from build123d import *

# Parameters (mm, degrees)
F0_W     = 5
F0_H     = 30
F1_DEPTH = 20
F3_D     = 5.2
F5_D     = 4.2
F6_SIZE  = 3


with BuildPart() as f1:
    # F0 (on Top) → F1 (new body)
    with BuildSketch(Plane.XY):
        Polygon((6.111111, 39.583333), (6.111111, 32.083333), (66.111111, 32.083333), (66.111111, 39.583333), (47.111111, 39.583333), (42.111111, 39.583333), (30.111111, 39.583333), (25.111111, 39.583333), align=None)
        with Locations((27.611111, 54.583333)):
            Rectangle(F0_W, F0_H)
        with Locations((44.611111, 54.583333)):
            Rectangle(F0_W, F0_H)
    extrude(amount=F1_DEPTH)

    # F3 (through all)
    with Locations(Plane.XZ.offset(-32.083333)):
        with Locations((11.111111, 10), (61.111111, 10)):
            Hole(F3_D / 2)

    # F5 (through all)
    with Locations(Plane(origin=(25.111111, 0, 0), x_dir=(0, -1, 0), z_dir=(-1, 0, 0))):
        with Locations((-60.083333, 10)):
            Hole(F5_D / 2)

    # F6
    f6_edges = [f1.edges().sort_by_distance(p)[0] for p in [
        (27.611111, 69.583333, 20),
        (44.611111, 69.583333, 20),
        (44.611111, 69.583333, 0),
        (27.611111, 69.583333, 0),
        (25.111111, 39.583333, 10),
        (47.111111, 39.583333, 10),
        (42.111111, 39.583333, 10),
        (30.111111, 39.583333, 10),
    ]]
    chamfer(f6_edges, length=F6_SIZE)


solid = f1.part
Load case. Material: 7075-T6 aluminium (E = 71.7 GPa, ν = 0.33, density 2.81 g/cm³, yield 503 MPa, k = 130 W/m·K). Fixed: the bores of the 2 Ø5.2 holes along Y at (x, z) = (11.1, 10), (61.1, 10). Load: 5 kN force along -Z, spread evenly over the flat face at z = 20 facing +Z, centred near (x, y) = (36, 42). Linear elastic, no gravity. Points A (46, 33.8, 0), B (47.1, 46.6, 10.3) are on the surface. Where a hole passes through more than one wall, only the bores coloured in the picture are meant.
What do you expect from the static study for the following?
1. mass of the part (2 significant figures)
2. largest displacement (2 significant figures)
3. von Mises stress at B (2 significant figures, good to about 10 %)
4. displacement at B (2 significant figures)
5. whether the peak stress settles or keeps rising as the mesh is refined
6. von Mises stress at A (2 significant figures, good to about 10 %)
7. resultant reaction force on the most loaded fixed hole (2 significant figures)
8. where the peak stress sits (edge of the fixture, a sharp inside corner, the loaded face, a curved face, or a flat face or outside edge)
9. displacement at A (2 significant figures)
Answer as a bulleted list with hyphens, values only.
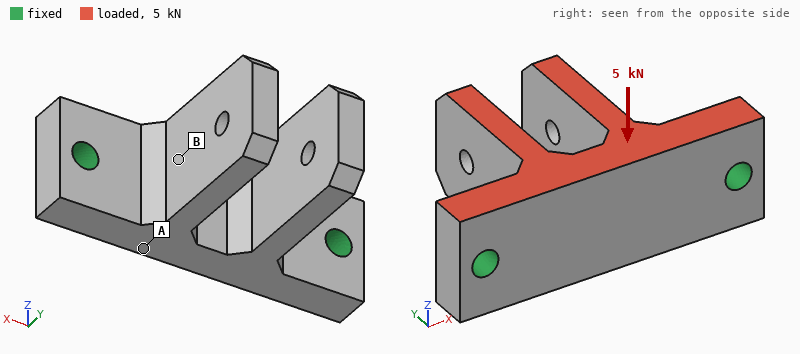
- 42 g
- 0.15 mm
- 22 MPa
- 0.055 mm
- keeps rising
- 47 MPa
- 2.5 kN
- edge of the fixture
- 0.033 mm
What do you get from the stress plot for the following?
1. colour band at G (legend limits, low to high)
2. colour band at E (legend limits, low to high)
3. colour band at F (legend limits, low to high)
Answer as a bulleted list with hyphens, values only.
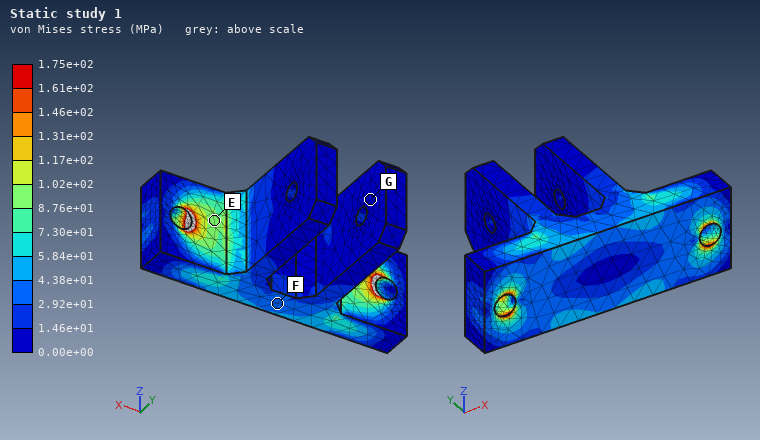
- 0.00e+00 to 1.46e+01 MPa
- 8.76e+01 to 1.02e+02 MPa
- 2.92e+01 to 4.38e+01 MPa
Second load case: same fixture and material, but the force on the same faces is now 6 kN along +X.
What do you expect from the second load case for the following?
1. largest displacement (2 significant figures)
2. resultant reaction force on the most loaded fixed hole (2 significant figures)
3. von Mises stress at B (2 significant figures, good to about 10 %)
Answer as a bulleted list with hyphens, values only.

- 0.23 mm
- 3.3 kN
- 110 MPa
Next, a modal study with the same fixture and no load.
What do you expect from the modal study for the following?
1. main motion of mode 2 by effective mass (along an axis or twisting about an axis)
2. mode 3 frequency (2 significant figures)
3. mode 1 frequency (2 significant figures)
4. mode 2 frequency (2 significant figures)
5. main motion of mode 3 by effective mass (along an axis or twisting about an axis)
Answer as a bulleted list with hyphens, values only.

- along X
- 5100 Hz
- 4400 Hz
- 4900 Hz
- along Z
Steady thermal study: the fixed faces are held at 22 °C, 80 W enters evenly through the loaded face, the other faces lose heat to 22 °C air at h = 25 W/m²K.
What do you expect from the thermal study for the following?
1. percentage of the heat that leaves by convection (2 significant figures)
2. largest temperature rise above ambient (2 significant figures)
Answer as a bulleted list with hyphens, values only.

- 4.1 %
- 42 K
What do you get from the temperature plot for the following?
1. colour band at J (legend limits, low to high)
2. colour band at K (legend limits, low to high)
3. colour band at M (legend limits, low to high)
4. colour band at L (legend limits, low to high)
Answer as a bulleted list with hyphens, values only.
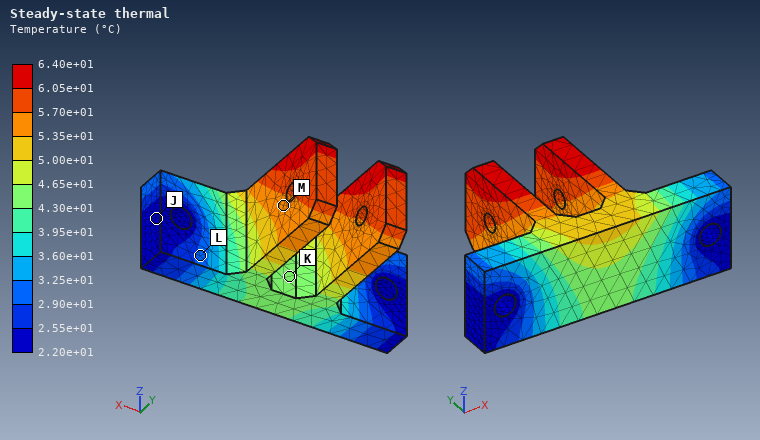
- 2.20e+01 to 2.55e+01 °C
- 4.30e+01 to 4.65e+01 °C
- 5.35e+01 to 5.70e+01 °C
- 2.90e+01 to 3.25e+01 °C
